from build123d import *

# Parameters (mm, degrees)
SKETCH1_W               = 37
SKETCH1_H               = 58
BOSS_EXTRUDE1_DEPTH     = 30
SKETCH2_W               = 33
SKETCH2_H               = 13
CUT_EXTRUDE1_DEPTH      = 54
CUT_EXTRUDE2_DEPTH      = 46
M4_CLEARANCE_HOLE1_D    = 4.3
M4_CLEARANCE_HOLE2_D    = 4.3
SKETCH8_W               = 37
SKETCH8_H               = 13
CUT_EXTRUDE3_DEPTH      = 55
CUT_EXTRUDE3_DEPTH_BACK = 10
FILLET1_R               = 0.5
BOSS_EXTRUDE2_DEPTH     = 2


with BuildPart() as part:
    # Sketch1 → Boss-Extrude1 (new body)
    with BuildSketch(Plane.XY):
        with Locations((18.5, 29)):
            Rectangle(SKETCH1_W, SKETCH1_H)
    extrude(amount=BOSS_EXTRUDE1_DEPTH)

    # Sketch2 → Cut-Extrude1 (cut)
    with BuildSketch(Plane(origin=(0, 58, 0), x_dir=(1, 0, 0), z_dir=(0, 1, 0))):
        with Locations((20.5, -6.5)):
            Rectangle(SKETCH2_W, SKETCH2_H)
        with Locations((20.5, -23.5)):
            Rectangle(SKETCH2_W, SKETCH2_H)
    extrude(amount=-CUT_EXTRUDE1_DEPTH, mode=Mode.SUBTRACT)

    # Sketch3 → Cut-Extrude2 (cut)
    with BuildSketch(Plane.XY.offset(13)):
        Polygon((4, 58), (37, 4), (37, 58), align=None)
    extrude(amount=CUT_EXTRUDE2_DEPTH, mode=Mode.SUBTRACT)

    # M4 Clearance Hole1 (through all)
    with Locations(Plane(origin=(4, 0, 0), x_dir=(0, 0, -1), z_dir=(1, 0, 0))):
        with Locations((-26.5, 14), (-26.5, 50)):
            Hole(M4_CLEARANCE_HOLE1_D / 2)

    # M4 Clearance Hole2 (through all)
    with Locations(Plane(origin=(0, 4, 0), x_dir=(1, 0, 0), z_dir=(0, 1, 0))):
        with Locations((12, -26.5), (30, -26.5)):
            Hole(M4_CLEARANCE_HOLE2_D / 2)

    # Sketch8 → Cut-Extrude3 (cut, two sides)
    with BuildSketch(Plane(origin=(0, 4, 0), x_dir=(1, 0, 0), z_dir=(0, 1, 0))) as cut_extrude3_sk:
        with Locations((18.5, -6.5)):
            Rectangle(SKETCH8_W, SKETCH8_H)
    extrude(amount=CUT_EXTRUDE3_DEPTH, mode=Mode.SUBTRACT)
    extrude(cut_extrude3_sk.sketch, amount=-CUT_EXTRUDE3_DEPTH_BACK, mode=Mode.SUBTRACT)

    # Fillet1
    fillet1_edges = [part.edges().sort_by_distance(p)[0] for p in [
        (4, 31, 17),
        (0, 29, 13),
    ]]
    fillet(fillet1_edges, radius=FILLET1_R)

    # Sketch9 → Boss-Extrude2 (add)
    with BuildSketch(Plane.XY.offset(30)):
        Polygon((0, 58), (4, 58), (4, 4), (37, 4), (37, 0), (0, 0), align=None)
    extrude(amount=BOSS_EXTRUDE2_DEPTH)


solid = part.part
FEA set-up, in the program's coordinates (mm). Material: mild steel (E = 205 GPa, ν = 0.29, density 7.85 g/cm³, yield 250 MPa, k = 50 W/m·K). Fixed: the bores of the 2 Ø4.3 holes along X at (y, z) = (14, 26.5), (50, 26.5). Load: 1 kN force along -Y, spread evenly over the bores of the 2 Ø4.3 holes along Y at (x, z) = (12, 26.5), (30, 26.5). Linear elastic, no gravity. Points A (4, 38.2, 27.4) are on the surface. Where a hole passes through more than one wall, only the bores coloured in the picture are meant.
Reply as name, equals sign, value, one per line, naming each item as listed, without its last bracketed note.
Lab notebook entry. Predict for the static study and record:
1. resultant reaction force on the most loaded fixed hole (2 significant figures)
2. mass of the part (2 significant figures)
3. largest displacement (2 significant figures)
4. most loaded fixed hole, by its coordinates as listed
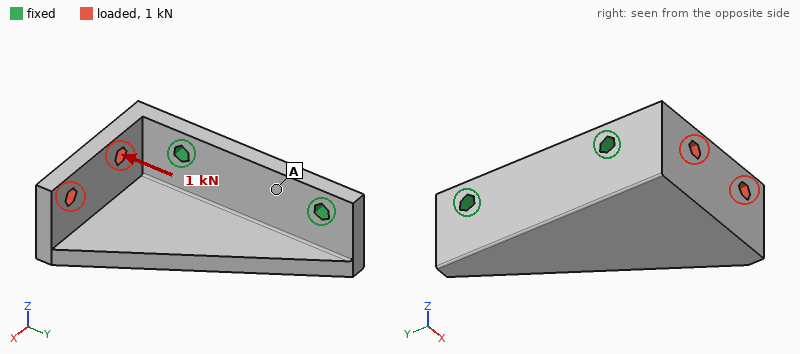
resultant reaction force on the most loaded fixed hole = 950 N
mass of the part = 80 g
largest displacement = 92 µm
most loaded fixed hole, by its coordinates as listed = (14, 26.5)
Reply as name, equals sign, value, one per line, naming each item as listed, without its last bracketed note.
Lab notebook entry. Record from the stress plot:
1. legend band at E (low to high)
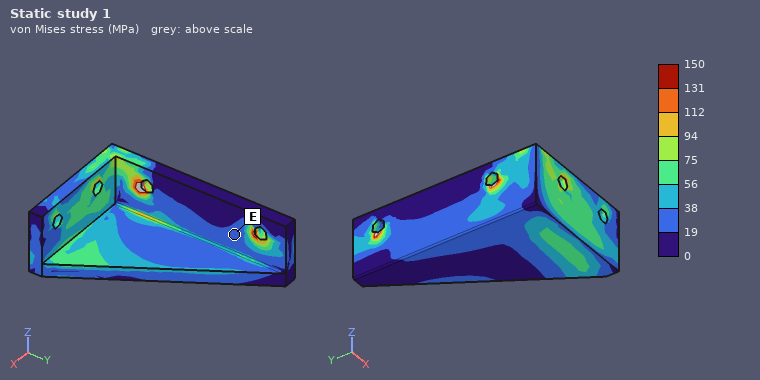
legend band at E = 19 to 38 MPa
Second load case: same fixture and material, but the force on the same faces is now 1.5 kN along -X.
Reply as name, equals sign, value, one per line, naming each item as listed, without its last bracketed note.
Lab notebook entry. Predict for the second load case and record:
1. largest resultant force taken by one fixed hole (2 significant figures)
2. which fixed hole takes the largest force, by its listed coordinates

largest resultant force taken by one fixed hole = 1.8 kN
which fixed hole takes the largest force, by its listed coordinates = (14, 26.5)
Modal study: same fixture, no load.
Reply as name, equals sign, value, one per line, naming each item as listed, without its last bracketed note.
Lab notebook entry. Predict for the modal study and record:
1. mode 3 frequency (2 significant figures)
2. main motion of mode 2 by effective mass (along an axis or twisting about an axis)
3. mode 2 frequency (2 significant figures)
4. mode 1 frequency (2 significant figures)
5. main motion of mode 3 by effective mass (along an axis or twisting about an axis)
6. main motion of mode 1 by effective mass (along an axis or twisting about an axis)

mode 3 frequency = 8300 Hz
main motion of mode 2 by effective mass = along Y
mode 2 frequency = 5400 Hz
mode 1 frequency = 2600 Hz
main motion of mode 3 by effective mass = along X
main motion of mode 1 by effective mass = along Z
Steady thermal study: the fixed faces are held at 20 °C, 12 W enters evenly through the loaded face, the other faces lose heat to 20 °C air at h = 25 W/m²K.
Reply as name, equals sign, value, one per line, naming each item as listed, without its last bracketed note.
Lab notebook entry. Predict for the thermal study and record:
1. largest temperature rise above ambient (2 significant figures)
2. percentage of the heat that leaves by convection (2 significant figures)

largest temperature rise above ambient = 57 K
percentage of the heat that leaves by convection = 22 %
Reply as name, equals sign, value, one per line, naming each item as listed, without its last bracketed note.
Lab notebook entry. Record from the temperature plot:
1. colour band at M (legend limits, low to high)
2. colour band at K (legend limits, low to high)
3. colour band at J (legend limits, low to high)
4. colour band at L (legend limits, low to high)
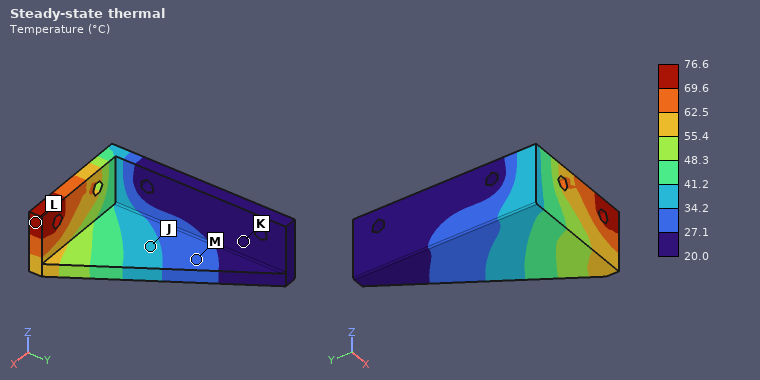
colour band at M = 27.1 to 34.2 °C
colour band at K = 20.0 to 27.1 °C
colour band at J = 34.2 to 41.2 °C
colour band at L = 69.6 to 76.6 °C
